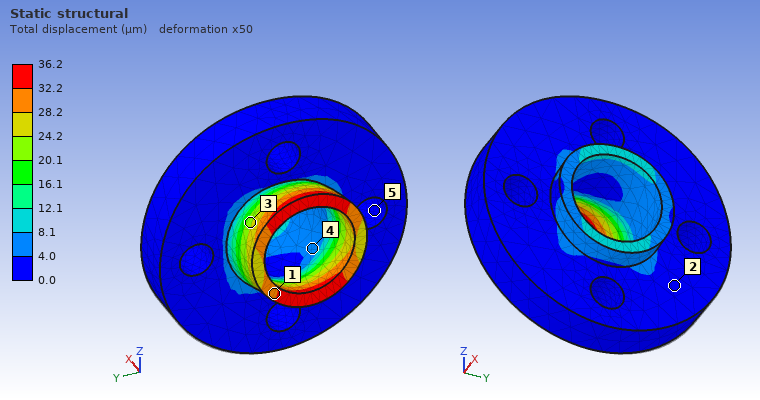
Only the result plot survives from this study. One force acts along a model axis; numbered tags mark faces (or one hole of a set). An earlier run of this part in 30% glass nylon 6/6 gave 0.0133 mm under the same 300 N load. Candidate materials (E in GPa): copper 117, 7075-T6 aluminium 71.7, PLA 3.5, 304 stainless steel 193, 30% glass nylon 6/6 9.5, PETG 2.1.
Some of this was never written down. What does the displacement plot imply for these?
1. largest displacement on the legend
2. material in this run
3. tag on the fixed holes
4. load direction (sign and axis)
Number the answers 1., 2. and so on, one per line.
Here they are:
1. 36.2 µm
2. PLA
3. 5
4. +Z
